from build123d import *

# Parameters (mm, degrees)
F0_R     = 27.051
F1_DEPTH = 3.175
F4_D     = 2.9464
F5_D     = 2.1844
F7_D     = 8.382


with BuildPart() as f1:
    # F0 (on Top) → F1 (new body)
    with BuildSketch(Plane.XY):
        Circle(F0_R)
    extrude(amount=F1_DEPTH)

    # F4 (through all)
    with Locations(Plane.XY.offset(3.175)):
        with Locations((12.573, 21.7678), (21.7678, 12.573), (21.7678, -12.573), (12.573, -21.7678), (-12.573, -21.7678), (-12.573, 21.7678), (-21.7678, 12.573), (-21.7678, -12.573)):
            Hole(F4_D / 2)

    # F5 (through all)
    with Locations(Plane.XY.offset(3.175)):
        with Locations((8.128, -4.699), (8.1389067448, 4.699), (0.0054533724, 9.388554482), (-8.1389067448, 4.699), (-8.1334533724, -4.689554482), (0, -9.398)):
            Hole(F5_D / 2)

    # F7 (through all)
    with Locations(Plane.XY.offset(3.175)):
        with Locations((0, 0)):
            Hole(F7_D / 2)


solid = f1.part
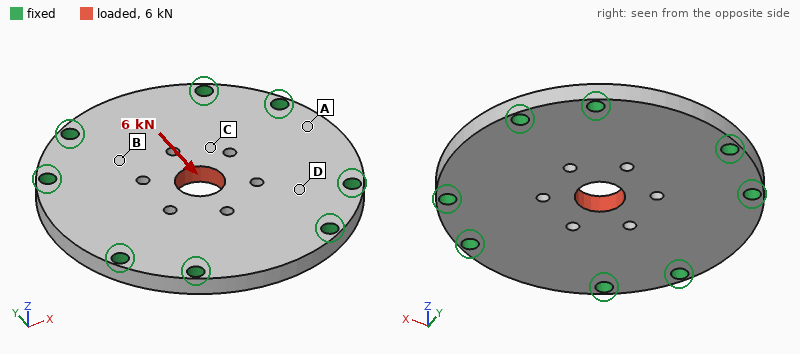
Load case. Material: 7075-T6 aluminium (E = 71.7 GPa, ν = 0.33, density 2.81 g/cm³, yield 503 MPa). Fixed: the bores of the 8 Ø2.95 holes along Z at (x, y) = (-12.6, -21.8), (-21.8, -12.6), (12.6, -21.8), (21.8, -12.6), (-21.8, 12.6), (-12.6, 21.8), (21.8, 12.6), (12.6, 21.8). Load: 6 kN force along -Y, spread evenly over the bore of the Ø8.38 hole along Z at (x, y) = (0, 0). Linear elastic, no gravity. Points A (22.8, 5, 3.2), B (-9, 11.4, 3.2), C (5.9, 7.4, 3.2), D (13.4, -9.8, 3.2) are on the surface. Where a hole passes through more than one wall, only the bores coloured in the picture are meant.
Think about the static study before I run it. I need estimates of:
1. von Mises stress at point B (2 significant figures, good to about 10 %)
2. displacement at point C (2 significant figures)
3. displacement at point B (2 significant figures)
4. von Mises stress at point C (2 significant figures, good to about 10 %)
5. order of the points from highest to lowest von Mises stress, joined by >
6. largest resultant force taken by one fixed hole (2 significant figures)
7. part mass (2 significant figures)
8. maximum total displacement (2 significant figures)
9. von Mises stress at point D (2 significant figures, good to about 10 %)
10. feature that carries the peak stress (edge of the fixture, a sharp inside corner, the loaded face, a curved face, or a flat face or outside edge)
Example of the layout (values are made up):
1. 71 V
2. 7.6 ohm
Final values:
1. 38 MPa
2. 9.4 µm
3. 5.8 µm
4. 47 MPa
5. C > B > D > A
6. 1.1 kN
7. 19 g
8. 16 µm
9. 23 MPa
10. a curved face
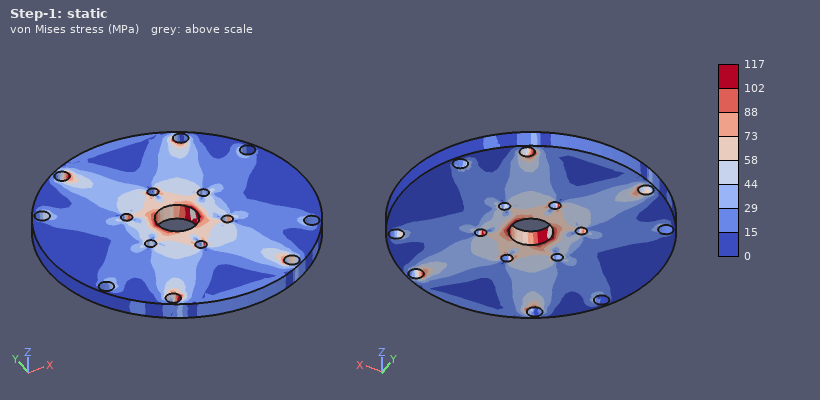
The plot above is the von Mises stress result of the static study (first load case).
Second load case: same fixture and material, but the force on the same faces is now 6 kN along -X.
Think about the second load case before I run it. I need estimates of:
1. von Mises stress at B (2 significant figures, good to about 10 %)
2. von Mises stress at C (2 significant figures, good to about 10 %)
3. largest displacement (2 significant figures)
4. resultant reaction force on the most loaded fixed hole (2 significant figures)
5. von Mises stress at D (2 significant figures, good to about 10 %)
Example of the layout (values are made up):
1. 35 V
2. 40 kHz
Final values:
1. 32 MPa
2. 41 MPa
3. 16 µm
4. 1.1 kN
5. 35 MPa
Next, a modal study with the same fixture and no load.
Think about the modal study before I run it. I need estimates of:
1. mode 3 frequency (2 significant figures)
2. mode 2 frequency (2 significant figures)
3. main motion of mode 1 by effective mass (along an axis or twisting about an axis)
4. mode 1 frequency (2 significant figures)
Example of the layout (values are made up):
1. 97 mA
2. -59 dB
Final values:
1. 20 kHz
2. 20 kHz
3. along Z
4. 11 kHz
